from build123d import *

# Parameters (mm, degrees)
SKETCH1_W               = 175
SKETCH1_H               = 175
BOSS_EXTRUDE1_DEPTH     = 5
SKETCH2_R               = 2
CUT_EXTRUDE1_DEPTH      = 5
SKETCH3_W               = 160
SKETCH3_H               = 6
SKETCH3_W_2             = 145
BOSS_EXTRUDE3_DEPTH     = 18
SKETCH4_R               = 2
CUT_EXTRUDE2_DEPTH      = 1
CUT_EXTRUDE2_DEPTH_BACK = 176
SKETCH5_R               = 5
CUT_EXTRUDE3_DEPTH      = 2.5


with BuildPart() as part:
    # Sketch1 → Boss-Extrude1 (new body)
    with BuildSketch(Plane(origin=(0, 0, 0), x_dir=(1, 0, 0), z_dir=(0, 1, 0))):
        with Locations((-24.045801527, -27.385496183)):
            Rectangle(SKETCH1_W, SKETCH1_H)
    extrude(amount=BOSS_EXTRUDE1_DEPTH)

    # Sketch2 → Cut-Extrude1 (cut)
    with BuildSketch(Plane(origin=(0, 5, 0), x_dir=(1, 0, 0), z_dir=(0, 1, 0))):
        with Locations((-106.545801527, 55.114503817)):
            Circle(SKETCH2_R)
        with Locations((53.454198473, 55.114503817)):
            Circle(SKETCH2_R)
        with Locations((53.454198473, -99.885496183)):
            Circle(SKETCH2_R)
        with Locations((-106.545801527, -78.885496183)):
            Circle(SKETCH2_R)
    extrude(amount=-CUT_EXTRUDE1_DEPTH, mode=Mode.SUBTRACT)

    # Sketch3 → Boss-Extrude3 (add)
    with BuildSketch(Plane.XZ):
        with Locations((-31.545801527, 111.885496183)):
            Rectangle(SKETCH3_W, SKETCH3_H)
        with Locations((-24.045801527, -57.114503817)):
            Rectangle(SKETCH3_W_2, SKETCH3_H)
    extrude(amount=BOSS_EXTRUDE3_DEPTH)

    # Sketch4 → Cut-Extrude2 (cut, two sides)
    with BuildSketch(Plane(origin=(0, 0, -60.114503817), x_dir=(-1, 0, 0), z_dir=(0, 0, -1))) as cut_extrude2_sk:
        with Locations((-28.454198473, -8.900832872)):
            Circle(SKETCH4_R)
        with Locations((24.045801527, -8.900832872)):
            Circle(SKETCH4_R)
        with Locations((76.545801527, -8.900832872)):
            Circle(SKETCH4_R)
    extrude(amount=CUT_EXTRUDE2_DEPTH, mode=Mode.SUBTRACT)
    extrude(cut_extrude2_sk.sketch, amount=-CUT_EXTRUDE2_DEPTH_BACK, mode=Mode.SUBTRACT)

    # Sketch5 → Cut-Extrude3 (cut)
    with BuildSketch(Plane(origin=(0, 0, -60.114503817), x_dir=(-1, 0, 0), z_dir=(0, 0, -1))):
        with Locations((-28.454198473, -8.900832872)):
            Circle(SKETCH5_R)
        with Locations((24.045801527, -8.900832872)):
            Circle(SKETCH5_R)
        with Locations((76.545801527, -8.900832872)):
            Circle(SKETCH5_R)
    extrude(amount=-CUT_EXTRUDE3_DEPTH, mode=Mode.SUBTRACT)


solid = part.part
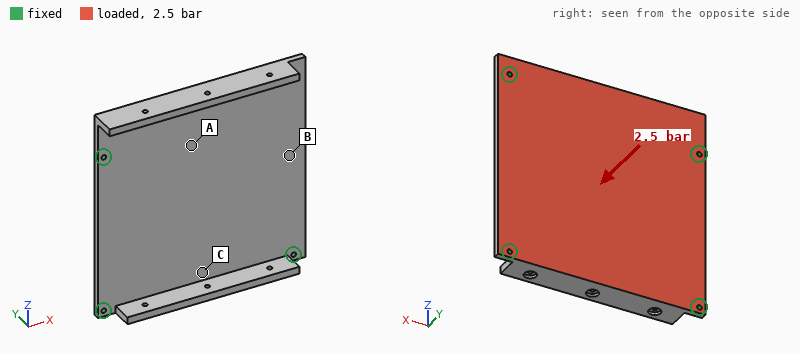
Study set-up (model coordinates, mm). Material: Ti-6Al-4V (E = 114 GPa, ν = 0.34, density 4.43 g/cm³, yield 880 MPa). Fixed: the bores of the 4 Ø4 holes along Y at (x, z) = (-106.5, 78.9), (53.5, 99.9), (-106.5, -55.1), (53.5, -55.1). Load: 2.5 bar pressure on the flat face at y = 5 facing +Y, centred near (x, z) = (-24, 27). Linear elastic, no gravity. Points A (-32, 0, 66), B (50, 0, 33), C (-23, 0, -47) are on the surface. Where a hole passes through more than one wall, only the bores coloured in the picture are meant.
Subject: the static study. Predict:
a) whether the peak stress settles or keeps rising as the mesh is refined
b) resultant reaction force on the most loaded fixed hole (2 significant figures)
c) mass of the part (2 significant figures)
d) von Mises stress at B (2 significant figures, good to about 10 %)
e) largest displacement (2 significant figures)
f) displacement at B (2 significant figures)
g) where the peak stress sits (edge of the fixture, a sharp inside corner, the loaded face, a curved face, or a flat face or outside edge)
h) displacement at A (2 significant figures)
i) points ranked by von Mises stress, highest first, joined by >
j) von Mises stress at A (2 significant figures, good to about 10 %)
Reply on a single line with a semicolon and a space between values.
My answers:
keeps rising; 2.4 kN; 820 g; 86 MPa; 0.69 mm; 0.54 mm; edge of the fixture; 0.46 mm; B > A > C; 48 MPa
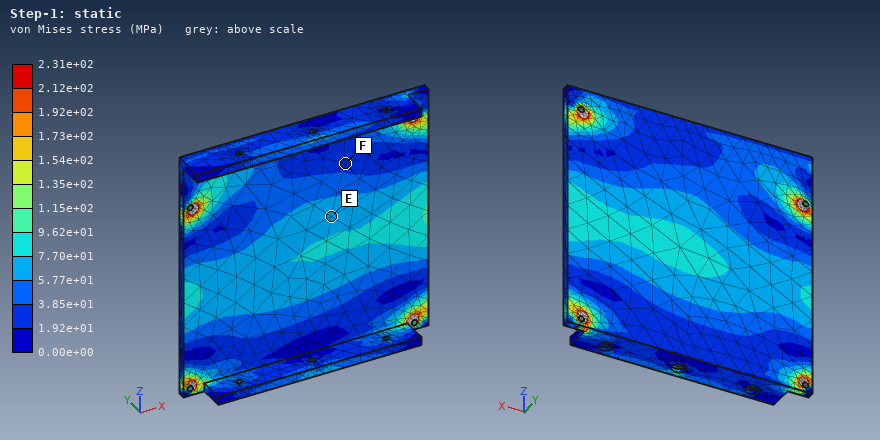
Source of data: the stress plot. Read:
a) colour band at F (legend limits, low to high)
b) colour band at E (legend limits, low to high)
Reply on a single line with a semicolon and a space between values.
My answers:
1.92e+01 to 3.85e+01 MPa; 5.77e+01 to 7.70e+01 MPa
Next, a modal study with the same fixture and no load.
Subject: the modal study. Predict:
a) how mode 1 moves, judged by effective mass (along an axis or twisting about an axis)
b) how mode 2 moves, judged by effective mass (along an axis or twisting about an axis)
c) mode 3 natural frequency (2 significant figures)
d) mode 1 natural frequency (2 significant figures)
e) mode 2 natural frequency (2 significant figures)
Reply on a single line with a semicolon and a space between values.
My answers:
along Y; along Y; 1300 Hz; 760 Hz; 1200 Hz
